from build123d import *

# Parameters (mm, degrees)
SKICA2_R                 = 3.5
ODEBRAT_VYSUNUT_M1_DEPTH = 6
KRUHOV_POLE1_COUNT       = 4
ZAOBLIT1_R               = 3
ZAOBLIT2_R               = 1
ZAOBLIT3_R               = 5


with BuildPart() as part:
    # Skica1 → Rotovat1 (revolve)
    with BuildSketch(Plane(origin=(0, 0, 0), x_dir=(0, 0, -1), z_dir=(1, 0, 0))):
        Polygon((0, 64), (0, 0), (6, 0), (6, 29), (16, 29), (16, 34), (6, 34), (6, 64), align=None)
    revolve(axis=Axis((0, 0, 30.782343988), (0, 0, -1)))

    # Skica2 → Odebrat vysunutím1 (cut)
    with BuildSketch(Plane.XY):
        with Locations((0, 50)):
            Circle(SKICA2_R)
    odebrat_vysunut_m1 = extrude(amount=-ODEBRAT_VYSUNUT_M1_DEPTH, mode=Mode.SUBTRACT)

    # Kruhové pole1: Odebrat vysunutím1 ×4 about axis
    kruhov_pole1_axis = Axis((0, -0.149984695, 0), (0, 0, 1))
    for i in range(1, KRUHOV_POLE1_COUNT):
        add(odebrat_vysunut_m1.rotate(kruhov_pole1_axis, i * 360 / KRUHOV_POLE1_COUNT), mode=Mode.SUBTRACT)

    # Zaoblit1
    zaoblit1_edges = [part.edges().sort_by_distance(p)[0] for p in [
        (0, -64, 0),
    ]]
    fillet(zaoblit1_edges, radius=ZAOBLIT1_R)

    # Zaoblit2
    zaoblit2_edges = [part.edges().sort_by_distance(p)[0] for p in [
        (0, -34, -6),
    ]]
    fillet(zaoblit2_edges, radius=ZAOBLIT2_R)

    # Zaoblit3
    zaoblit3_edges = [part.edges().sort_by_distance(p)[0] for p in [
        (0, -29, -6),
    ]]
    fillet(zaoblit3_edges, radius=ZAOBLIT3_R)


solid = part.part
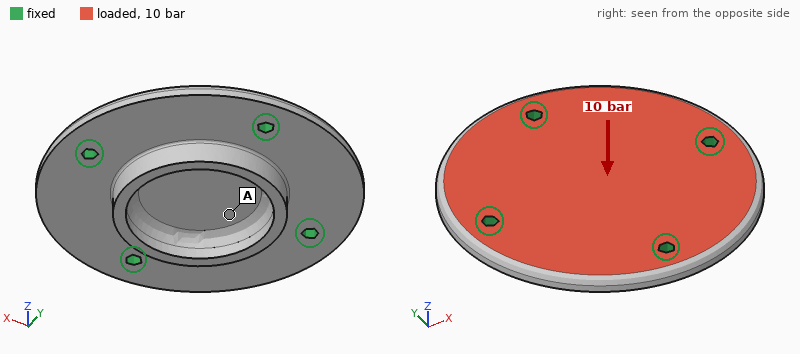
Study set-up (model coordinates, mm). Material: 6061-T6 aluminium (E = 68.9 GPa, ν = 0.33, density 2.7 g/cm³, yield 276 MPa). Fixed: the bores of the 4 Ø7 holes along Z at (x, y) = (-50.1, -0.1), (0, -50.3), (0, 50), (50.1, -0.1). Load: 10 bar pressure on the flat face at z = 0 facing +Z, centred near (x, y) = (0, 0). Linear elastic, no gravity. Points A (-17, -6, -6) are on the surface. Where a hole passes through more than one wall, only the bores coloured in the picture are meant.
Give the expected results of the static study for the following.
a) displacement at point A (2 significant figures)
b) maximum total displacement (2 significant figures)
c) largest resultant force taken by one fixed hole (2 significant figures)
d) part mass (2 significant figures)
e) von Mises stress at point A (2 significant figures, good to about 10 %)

56 µm
75 µm
2.9 kN
230 g
12 MPa
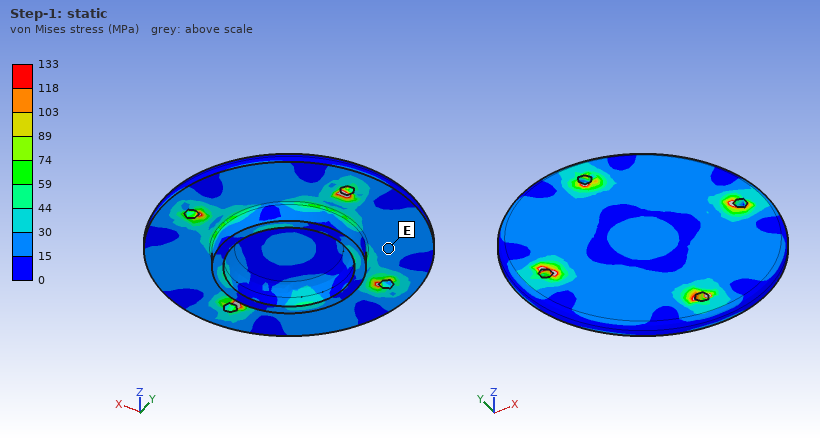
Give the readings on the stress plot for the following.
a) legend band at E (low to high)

15 to 30 MPa
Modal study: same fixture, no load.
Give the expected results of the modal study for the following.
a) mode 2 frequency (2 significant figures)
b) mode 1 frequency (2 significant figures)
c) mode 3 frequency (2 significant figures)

5000 Hz
4700 Hz
5000 Hz
